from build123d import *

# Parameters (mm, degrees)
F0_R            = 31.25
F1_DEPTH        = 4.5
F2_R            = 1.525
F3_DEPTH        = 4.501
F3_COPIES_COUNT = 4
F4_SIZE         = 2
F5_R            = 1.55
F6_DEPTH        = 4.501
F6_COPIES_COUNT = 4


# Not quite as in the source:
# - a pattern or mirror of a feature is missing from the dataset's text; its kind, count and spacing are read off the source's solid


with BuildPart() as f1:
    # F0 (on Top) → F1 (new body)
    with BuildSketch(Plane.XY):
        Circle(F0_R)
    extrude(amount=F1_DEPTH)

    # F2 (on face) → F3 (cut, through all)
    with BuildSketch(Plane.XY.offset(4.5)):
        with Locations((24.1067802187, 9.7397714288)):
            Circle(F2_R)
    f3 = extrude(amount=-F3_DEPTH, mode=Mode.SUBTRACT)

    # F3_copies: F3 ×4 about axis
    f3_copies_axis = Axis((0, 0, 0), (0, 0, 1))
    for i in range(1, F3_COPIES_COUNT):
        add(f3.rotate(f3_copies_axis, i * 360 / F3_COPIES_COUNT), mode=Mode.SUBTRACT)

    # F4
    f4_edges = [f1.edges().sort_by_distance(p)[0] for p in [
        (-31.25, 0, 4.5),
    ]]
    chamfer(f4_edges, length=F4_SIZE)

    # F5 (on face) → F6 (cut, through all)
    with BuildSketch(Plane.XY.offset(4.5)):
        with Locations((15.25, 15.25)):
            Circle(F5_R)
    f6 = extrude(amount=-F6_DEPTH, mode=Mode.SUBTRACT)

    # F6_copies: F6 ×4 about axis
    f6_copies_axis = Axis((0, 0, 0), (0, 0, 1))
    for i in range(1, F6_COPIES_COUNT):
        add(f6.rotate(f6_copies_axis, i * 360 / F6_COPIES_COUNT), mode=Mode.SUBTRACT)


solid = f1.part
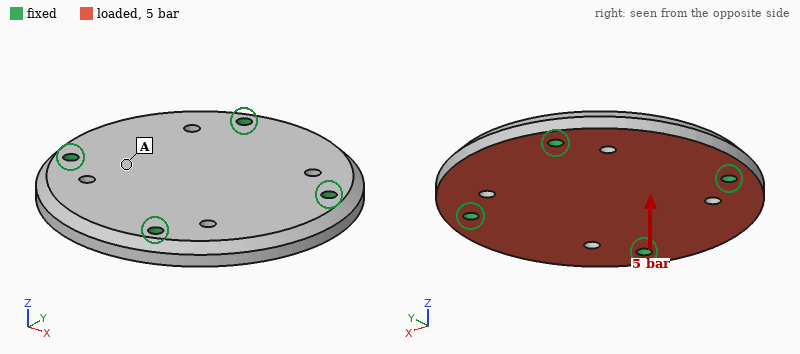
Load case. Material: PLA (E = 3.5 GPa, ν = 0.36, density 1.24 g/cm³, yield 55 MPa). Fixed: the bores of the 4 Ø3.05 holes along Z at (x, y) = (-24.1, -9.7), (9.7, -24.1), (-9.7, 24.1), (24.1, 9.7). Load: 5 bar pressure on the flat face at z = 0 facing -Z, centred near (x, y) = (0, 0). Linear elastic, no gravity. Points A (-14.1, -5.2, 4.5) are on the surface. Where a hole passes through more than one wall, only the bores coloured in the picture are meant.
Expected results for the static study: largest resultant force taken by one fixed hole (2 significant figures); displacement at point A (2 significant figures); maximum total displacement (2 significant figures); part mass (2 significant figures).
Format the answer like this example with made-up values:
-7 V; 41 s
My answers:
380 N; 0.14 mm; 0.23 mm; 16 g
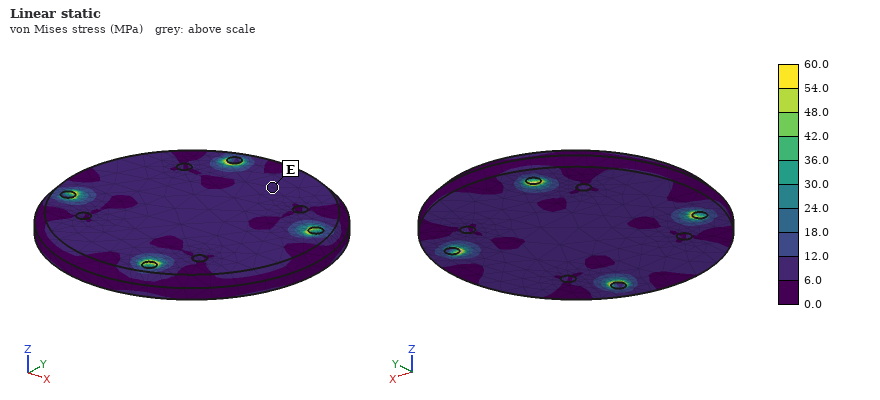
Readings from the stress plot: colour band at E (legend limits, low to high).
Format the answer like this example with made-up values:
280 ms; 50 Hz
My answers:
6.0 to 12.0 MPa
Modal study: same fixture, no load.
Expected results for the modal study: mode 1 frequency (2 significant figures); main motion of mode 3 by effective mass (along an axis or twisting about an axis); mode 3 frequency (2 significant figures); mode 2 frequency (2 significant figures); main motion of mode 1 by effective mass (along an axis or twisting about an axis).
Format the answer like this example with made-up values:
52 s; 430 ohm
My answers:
3700 Hz; twisting about X; 4300 Hz; 4000 Hz; along Z
